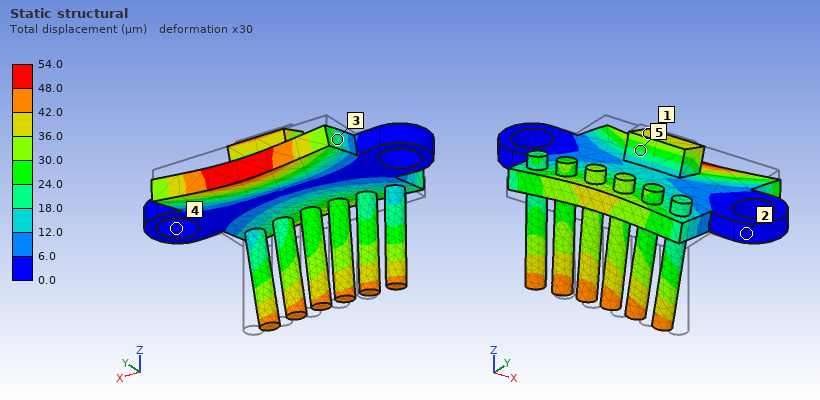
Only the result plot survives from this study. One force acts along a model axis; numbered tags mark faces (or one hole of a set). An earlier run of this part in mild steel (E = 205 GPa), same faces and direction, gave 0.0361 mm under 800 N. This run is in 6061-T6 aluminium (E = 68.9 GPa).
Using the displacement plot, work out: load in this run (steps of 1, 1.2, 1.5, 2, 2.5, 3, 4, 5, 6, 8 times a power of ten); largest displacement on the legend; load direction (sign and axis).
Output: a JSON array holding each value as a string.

["400 N", "54.0 µm", "+Y"]
